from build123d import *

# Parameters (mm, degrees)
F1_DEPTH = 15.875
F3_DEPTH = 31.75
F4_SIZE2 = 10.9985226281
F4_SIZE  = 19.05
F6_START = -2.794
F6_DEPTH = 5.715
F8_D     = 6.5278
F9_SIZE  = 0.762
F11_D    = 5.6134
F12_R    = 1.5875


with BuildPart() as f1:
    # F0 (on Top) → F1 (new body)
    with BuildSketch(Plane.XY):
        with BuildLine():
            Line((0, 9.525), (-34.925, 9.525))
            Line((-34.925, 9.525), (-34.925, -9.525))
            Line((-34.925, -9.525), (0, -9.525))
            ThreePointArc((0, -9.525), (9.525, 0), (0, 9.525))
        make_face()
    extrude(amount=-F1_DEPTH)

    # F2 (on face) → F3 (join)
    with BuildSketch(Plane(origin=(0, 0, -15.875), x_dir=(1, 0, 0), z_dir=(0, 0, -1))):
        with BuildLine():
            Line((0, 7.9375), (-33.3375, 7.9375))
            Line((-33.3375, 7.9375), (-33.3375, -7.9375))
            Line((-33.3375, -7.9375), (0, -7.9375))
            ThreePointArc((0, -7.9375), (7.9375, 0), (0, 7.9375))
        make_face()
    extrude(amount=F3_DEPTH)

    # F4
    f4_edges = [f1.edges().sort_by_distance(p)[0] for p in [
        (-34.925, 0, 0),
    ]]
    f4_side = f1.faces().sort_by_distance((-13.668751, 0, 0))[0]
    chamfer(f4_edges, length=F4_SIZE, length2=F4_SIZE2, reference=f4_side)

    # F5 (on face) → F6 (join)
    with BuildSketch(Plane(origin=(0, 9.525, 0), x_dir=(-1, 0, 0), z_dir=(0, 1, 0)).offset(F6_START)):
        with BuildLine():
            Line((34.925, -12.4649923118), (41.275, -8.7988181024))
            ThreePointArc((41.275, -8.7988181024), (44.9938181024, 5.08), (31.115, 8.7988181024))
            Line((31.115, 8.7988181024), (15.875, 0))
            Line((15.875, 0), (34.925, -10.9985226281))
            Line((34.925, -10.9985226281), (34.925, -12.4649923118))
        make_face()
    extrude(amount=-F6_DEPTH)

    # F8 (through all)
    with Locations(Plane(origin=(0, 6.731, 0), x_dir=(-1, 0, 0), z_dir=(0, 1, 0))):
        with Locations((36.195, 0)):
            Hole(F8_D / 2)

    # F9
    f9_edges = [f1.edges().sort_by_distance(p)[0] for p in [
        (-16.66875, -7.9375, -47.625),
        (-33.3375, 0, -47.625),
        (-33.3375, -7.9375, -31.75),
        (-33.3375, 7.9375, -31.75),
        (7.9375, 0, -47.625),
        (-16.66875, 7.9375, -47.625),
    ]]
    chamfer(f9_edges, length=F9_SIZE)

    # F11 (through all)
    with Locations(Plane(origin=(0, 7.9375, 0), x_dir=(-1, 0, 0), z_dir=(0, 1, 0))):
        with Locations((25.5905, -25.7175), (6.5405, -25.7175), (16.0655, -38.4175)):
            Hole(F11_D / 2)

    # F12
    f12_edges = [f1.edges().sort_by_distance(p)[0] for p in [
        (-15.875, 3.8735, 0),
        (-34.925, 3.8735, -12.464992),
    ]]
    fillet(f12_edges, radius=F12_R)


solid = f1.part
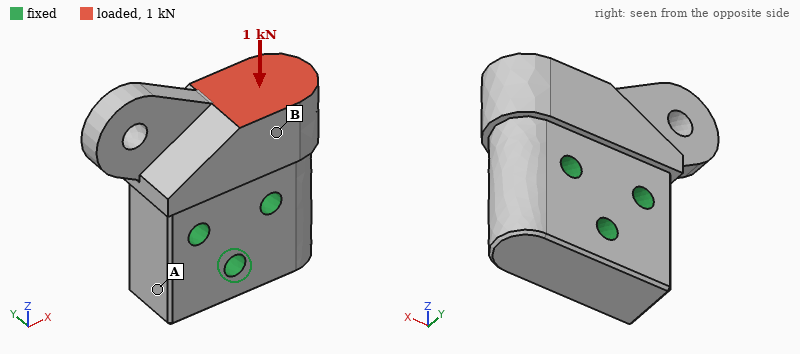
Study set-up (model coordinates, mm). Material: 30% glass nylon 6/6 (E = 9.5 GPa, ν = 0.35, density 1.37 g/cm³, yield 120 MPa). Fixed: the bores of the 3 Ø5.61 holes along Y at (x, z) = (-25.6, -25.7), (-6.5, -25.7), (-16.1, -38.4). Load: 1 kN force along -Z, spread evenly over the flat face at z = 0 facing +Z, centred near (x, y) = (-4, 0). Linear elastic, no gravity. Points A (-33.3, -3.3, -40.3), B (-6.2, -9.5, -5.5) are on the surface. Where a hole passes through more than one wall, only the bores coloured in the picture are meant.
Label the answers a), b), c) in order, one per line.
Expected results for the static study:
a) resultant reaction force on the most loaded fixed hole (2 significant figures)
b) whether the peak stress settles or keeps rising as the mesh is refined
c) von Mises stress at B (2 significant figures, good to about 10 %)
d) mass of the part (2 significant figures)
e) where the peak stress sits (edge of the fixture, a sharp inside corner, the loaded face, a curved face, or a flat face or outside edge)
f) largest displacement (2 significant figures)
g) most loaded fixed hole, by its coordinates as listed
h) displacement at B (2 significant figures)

a) 920 N
b) keeps rising
c) 2.4 MPa
d) 43 g
e) edge of the fixture
f) 14 µm
g) (-6.5, -25.7)
h) 7.8 µm
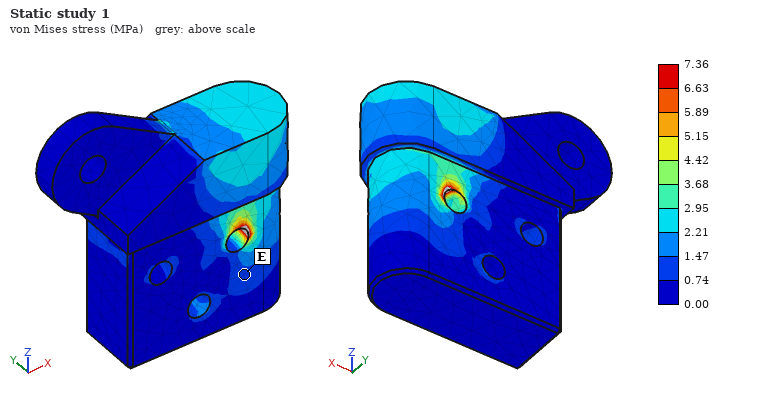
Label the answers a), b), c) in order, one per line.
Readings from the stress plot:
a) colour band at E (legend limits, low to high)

a) 0.74 to 1.47 MPa
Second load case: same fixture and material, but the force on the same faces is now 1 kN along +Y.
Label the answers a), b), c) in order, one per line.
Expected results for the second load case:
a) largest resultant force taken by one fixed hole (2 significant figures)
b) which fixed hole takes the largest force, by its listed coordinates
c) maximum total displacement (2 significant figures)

a) 950 N
b) (-6.5, -25.7)
c) 88 µm
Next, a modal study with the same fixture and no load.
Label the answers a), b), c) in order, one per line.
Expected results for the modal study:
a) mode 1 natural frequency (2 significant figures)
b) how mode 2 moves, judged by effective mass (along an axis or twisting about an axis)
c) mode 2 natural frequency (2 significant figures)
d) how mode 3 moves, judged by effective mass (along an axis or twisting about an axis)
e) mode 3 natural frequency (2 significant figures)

a) 4800 Hz
b) along Y
c) 7600 Hz
d) along X
e) 8600 Hz
